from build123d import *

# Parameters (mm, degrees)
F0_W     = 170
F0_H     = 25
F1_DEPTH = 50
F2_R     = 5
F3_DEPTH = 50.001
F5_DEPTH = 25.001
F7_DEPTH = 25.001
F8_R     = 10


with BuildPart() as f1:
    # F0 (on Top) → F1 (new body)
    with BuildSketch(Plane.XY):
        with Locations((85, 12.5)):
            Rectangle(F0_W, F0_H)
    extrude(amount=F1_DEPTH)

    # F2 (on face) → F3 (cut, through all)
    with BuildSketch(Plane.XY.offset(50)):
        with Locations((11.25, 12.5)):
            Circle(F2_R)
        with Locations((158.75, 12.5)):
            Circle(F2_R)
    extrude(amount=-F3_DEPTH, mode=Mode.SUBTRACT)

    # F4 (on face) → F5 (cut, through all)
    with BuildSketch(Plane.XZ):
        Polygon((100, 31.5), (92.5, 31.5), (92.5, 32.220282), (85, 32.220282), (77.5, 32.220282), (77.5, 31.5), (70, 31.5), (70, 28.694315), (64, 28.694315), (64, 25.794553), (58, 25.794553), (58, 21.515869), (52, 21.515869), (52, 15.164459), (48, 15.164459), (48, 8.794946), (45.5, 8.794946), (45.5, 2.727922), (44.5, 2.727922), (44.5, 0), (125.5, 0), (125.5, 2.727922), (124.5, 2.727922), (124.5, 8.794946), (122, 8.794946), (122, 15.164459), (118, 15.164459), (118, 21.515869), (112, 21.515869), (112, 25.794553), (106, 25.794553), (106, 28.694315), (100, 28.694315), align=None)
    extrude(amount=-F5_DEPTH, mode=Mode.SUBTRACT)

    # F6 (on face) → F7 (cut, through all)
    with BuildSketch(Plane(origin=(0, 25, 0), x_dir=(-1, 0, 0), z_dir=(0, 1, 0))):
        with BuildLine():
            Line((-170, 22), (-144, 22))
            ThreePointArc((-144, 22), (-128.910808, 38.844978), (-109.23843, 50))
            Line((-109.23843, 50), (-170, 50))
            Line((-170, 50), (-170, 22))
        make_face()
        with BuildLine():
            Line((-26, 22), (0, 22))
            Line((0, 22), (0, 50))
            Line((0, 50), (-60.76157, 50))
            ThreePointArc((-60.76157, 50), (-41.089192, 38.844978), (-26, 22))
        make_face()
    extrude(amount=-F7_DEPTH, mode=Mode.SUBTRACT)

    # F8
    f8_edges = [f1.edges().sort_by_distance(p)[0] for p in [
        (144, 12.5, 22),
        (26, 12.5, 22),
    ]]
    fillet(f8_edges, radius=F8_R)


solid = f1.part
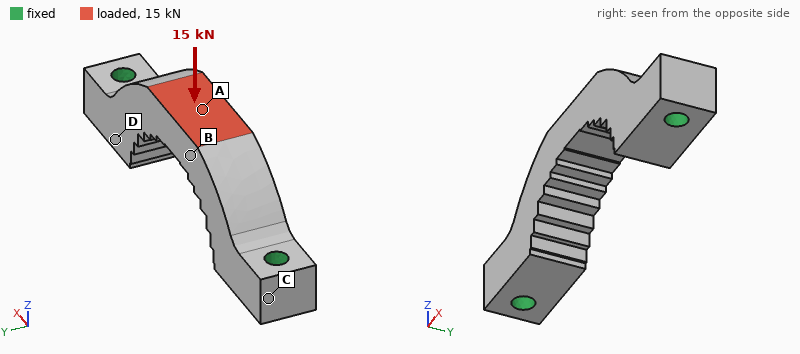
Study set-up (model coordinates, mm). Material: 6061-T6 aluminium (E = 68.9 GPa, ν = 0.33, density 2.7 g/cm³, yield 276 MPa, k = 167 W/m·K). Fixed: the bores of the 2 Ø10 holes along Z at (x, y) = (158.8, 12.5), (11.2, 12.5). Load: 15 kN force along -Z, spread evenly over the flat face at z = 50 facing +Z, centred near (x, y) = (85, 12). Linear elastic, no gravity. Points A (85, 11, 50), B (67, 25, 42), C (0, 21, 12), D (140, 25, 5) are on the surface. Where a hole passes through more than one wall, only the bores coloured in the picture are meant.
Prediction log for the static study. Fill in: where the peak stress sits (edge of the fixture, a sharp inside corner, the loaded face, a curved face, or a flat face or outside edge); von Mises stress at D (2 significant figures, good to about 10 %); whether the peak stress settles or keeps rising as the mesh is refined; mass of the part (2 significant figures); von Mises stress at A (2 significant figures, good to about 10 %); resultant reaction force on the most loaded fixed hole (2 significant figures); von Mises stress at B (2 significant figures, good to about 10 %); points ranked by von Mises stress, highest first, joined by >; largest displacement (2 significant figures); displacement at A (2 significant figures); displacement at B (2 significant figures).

edge of the fixture
20 MPa
keeps rising
280 g
58 MPa
12 kN
32 MPa
A > B > D > C
68 µm
66 µm
55 µm
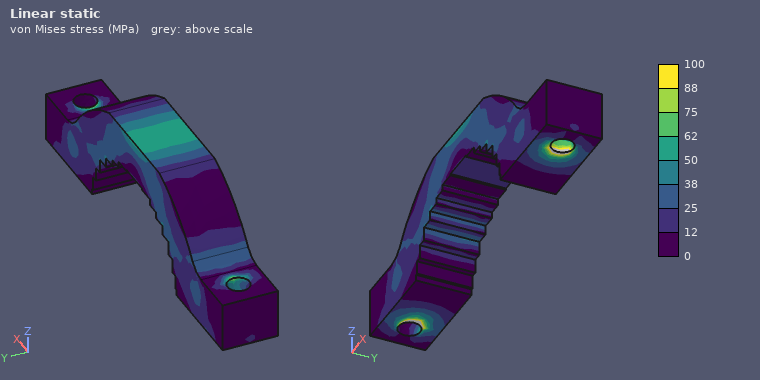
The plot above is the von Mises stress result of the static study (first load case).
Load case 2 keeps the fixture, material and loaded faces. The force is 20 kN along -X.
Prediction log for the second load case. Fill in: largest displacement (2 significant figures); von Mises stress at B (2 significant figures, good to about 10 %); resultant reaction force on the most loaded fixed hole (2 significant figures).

34 µm
19 MPa
11 kN
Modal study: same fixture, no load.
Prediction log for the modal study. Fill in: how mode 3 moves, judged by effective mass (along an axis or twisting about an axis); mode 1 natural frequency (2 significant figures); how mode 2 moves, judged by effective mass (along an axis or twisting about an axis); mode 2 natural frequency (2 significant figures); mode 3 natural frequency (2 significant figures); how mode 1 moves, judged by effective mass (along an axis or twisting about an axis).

along X
3400 Hz
along Z
7600 Hz
8500 Hz
along Y
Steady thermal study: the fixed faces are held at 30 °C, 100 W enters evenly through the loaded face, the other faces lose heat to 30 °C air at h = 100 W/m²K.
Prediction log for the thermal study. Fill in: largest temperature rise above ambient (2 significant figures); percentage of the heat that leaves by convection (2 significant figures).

35 K
23 %
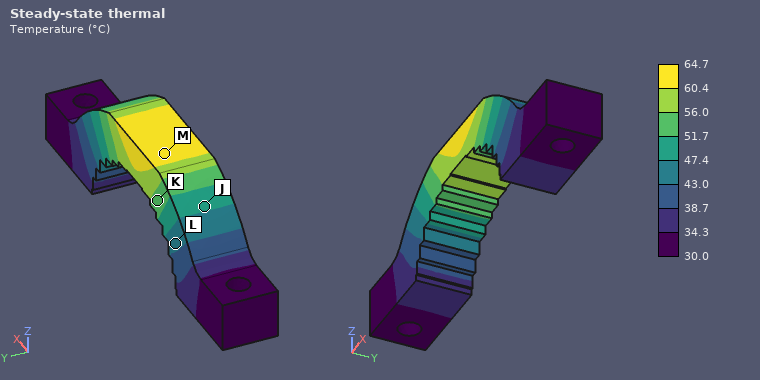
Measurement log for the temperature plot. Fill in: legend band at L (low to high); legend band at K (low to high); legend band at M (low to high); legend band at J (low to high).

43.0 to 47.4 °C
51.7 to 56.0 °C
60.4 to 64.7 °C
47.4 to 51.7 °C
